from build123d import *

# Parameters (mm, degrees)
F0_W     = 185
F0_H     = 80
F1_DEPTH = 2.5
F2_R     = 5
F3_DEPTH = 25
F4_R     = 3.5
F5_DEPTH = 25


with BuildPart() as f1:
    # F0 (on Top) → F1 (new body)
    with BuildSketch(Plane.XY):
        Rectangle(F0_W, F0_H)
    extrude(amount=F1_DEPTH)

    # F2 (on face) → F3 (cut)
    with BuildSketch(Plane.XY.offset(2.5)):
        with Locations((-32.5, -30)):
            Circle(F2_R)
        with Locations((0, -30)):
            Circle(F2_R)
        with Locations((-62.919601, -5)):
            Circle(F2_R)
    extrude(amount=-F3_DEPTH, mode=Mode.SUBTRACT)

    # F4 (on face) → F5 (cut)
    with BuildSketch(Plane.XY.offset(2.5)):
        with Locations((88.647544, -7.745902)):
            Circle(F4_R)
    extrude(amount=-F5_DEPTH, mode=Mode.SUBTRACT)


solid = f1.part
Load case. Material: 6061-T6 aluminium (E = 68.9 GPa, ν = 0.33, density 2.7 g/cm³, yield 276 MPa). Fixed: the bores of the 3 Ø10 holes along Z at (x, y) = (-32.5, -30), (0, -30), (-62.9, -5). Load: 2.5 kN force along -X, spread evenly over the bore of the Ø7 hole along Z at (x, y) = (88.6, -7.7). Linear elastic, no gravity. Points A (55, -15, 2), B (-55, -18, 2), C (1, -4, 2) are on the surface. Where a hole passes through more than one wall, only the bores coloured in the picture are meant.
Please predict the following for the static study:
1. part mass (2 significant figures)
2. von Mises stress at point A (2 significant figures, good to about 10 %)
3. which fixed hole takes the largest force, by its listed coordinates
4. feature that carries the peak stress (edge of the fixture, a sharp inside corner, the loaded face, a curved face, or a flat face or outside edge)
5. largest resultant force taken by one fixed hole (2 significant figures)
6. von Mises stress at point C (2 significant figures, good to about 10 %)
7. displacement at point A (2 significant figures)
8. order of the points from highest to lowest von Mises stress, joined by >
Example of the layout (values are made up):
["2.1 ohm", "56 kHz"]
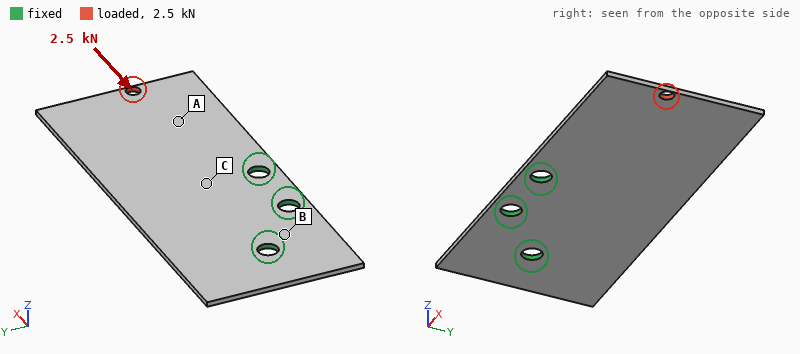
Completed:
["98 g", "22 MPa", "(0, -30)", "the loaded face", "1.5 kN", "12 MPa", "20 µm", "A > C > B"]
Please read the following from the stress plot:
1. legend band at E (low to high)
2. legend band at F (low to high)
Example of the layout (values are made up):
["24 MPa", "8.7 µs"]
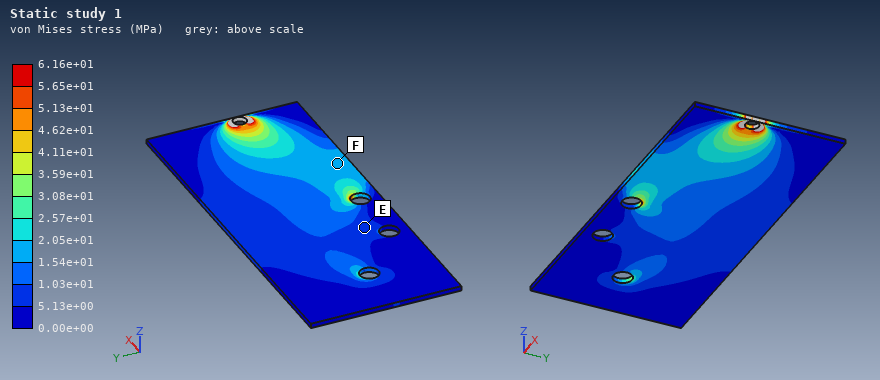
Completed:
["5.13e+00 to 1.03e+01 MPa", "1.54e+01 to 2.05e+01 MPa"]
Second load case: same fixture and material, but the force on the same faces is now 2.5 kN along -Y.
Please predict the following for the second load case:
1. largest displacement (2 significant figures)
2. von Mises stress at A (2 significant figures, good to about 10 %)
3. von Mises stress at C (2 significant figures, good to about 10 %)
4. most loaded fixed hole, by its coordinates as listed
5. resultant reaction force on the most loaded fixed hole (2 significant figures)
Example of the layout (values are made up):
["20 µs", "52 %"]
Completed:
["0.25 mm", "28 MPa", "34 MPa", "(0, -30)", "5.3 kN"]
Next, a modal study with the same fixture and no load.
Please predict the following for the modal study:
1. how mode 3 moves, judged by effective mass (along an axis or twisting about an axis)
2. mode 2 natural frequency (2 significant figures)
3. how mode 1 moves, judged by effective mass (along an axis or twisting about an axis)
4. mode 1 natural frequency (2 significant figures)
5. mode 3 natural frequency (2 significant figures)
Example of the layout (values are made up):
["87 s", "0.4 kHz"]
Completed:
["along Z", "460 Hz", "along Z", "200 Hz", "880 Hz"]
